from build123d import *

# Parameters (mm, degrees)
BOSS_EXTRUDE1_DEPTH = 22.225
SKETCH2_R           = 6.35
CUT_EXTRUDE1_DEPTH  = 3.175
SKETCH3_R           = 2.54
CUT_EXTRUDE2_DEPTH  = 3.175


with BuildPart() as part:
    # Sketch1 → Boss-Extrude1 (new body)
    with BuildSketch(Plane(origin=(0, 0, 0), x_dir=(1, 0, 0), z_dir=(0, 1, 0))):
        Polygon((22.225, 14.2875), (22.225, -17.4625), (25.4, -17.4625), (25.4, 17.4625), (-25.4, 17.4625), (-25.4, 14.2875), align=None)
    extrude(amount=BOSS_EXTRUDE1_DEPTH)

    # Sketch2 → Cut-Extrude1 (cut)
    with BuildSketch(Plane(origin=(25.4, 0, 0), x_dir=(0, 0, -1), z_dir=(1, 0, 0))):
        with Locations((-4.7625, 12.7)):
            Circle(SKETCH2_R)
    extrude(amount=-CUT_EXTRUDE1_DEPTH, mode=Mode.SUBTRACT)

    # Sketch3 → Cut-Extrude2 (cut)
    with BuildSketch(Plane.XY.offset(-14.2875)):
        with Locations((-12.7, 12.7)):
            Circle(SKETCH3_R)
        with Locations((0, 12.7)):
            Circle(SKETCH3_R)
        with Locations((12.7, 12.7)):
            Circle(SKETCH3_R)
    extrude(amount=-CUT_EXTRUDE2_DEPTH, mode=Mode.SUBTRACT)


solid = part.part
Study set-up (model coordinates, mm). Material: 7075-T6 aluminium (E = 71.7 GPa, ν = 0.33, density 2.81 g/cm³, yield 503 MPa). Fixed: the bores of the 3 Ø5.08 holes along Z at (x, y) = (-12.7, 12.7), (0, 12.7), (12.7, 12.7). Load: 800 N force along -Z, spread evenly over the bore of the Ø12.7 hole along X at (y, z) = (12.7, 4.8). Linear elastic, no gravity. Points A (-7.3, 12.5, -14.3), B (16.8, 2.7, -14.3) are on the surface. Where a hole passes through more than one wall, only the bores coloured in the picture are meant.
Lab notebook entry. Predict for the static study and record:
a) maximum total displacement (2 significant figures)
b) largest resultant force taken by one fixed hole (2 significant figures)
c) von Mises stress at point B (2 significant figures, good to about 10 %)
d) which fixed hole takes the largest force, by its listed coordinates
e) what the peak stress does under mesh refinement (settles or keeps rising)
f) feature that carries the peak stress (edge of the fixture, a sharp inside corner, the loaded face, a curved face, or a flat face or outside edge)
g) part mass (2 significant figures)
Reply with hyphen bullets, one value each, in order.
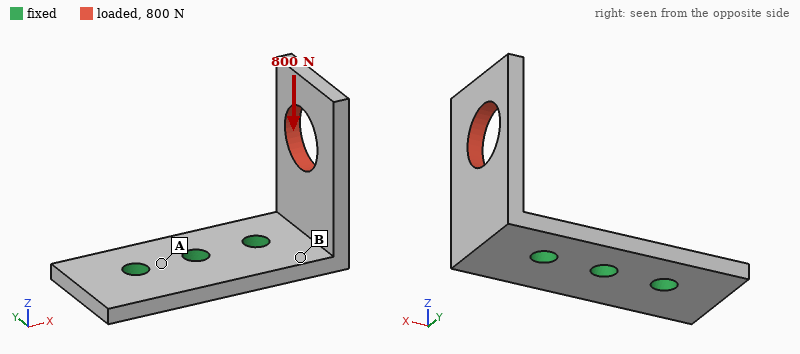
- 0.35 mm
- 940 N
- 83 MPa
- (12.7, 12.7)
- keeps rising
- edge of the fixture
- 15 g
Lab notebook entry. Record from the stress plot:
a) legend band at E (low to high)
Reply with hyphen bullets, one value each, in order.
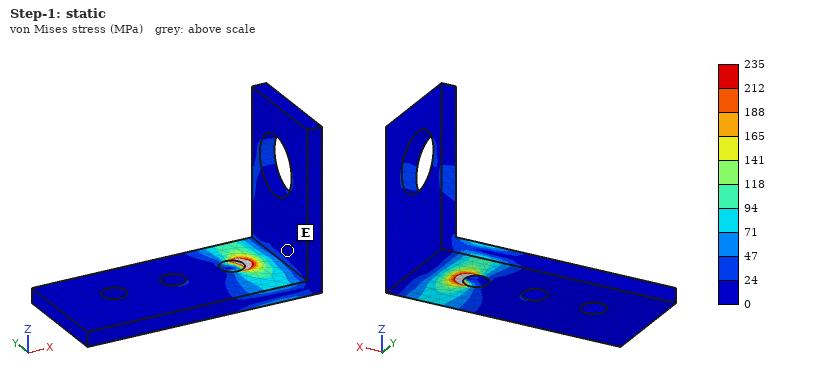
- 0 to 24 MPa
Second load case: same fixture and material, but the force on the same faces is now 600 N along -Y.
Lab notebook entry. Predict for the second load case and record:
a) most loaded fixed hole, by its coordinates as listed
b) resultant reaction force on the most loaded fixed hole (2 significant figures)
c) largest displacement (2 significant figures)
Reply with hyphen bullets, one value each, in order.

- (12.7, 12.7)
- 820 N
- 0.59 mm
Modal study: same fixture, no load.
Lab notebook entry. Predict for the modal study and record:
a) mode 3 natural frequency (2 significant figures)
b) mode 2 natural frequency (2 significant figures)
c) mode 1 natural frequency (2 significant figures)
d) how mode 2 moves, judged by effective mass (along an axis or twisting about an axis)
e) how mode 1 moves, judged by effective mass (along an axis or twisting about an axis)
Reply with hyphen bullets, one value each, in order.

- 6400 Hz
- 2900 Hz
- 1700 Hz
- along Y
- along X
